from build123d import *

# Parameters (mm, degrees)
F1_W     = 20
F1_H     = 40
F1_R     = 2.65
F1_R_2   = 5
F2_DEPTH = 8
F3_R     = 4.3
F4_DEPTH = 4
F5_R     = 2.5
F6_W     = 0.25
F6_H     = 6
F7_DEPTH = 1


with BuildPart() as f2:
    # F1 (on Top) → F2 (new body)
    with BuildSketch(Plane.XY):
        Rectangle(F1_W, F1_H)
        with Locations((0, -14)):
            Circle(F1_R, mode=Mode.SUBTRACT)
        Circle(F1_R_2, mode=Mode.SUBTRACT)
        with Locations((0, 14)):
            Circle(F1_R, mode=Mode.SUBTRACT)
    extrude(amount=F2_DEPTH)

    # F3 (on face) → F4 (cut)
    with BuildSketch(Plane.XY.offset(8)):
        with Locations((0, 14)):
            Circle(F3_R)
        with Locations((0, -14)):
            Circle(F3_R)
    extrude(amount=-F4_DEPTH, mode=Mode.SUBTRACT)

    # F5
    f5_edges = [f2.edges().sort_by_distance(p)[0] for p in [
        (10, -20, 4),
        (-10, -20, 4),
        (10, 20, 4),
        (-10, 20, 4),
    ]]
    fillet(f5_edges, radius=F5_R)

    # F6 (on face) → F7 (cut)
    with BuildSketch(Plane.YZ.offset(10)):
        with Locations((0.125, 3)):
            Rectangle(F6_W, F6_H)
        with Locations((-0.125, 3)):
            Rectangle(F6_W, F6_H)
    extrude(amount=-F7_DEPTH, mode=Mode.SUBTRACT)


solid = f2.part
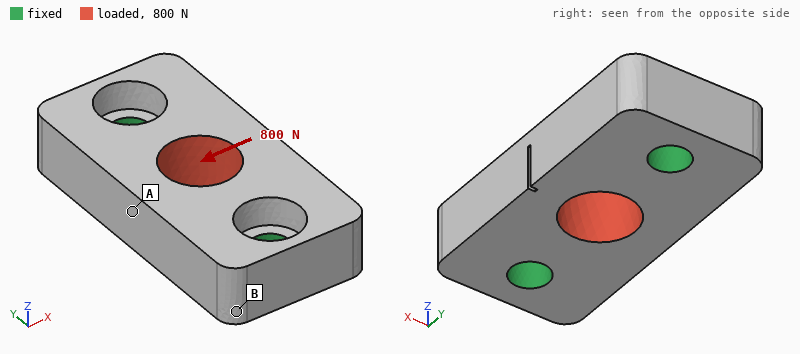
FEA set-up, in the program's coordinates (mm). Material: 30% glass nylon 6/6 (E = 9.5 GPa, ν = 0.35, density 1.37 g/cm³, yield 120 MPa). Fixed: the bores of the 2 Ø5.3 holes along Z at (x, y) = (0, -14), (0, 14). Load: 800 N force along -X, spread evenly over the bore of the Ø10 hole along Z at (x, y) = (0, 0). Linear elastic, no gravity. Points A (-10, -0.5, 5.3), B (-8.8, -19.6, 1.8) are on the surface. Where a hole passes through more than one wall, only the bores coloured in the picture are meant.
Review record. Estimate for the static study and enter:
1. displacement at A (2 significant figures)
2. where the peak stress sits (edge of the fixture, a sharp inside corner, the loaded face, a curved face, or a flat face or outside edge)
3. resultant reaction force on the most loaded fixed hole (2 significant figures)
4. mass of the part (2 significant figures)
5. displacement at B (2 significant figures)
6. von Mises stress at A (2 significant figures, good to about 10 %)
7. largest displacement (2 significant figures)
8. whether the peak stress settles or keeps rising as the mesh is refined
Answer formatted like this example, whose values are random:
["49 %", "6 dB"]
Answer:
["25 µm", "edge of the fixture", "400 N", "7.0 g", "9.5 µm", "9.4 MPa", "30 µm", "keeps rising"]
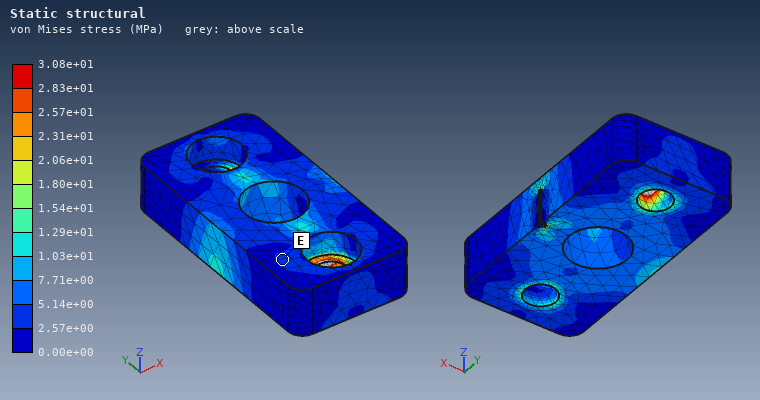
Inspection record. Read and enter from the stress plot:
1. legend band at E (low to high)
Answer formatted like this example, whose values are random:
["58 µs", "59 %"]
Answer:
["2.57e+00 to 5.14e+00 MPa"]
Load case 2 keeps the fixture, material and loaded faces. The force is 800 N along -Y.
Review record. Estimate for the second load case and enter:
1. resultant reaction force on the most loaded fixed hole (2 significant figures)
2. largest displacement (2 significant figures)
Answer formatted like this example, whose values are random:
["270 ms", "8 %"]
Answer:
["400 N", "8.0 µm"]
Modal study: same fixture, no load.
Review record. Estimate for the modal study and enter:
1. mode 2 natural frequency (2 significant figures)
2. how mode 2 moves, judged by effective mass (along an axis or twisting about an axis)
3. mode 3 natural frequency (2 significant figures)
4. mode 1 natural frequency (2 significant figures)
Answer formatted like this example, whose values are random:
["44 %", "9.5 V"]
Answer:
["14 kHz", "along Z", "17 kHz", "10 kHz"]
